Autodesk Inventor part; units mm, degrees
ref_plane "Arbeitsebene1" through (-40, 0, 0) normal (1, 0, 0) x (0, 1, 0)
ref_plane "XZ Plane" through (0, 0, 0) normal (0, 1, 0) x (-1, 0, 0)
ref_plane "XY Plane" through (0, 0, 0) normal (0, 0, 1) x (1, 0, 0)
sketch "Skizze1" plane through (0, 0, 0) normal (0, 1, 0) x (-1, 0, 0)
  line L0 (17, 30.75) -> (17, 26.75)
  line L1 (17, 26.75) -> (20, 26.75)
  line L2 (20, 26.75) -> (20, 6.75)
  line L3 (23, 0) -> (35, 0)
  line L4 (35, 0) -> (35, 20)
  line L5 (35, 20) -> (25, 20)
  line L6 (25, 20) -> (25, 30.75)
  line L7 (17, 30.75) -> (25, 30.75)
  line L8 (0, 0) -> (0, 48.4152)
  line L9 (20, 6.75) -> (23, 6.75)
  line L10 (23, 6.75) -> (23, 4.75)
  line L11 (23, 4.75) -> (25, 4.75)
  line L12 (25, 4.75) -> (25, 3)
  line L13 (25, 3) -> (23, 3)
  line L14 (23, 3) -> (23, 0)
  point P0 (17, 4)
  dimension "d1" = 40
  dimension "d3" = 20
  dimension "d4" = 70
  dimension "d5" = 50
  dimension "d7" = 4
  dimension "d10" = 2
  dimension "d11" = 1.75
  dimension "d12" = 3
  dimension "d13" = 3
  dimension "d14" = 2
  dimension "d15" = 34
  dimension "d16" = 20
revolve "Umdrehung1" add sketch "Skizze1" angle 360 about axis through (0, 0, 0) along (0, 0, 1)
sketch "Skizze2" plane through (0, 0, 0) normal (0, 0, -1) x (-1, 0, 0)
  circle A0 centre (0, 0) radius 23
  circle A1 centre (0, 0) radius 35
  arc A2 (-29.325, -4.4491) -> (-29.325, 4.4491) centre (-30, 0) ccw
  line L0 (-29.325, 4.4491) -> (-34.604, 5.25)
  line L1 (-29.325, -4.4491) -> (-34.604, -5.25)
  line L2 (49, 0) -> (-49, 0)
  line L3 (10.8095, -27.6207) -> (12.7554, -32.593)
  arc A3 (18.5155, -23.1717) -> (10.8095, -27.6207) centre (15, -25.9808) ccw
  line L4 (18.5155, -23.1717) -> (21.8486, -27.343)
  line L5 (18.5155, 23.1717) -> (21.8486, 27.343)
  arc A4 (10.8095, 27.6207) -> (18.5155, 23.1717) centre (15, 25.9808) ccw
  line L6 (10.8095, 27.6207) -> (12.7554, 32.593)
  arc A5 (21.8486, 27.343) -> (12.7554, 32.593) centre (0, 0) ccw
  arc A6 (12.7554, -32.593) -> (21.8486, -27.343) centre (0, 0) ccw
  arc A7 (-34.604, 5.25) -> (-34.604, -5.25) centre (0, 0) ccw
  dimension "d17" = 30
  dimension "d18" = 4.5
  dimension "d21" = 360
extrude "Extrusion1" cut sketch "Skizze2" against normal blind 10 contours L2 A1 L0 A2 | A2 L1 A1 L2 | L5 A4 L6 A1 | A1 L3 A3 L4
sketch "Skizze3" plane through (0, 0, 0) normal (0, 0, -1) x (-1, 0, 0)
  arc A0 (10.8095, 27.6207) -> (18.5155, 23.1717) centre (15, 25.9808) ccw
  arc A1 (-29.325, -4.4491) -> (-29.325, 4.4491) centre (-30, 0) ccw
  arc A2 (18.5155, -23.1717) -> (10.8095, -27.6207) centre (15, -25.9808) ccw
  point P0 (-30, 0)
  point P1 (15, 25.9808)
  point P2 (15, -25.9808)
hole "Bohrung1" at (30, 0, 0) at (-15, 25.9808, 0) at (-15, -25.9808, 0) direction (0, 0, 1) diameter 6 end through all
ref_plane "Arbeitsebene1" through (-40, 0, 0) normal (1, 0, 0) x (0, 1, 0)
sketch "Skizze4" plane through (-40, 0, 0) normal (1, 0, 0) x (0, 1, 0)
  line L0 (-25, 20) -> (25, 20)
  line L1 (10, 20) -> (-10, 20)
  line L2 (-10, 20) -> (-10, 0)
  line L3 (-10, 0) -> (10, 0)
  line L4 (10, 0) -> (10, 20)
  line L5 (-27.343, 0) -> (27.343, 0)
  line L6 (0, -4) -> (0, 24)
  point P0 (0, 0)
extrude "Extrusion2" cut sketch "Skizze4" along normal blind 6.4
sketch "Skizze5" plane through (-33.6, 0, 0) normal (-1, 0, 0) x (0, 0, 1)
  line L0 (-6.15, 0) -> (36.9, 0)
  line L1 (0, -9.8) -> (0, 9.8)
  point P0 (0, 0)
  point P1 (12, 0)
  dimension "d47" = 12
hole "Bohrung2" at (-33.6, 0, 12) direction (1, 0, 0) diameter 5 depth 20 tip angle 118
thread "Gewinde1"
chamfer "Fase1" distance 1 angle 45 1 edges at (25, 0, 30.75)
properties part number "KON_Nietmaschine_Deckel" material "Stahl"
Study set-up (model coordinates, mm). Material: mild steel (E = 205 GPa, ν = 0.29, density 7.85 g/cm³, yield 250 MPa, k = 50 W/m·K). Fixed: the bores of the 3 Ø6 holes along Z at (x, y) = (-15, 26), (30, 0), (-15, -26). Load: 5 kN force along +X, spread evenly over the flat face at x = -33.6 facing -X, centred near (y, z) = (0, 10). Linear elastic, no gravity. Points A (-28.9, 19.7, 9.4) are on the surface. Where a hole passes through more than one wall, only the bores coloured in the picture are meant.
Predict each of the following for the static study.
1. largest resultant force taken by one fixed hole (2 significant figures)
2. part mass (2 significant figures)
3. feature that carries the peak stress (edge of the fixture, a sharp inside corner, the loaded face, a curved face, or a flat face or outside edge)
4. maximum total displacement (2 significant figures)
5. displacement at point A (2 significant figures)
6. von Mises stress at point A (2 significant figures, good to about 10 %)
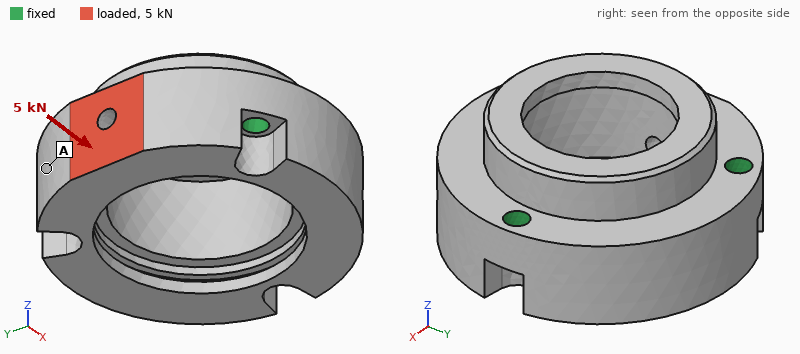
3.3 kN
420 g
edge of the fixture
9.2 µm
2.9 µm
7.9 MPa
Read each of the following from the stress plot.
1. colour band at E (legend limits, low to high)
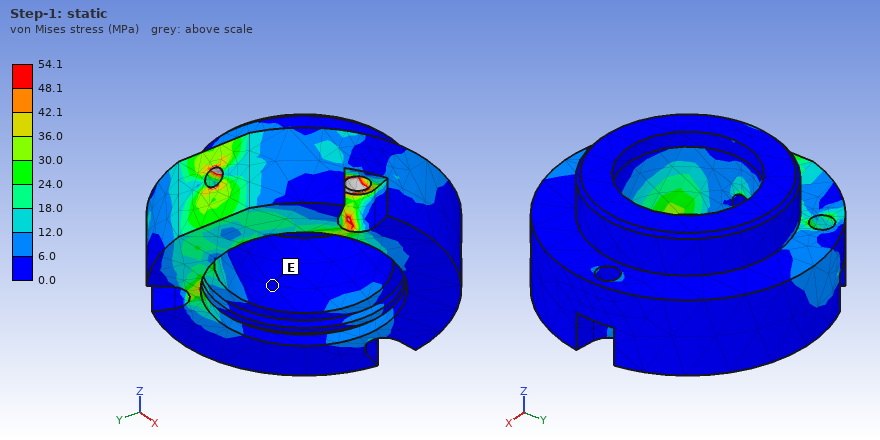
0.0 to 6.0 MPa
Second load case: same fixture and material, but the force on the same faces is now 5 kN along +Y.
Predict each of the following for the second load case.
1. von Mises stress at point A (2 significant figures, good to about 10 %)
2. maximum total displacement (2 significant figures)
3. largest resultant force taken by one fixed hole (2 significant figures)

12 MPa
3.1 µm
3.1 kN
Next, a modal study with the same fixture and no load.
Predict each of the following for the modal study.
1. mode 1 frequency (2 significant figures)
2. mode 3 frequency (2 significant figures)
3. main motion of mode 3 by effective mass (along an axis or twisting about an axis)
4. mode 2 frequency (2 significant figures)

11 kHz
16 kHz
along Z
11 kHz
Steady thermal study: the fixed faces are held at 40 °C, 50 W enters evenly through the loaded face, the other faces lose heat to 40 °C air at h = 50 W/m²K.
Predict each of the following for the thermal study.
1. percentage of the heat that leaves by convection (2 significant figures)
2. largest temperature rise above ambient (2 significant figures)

15 %
56 K
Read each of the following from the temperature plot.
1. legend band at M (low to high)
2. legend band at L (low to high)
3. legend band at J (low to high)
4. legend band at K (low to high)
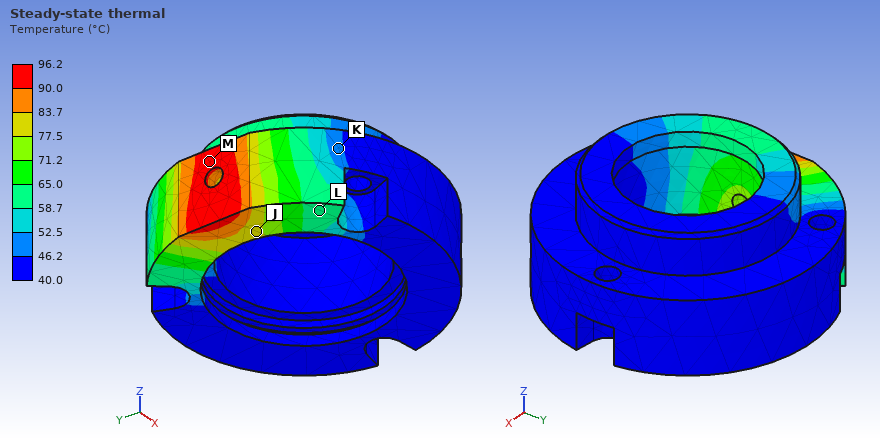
90.0 to 96.2 °C
58.7 to 65.0 °C
77.5 to 83.7 °C
46.2 to 52.5 °C
